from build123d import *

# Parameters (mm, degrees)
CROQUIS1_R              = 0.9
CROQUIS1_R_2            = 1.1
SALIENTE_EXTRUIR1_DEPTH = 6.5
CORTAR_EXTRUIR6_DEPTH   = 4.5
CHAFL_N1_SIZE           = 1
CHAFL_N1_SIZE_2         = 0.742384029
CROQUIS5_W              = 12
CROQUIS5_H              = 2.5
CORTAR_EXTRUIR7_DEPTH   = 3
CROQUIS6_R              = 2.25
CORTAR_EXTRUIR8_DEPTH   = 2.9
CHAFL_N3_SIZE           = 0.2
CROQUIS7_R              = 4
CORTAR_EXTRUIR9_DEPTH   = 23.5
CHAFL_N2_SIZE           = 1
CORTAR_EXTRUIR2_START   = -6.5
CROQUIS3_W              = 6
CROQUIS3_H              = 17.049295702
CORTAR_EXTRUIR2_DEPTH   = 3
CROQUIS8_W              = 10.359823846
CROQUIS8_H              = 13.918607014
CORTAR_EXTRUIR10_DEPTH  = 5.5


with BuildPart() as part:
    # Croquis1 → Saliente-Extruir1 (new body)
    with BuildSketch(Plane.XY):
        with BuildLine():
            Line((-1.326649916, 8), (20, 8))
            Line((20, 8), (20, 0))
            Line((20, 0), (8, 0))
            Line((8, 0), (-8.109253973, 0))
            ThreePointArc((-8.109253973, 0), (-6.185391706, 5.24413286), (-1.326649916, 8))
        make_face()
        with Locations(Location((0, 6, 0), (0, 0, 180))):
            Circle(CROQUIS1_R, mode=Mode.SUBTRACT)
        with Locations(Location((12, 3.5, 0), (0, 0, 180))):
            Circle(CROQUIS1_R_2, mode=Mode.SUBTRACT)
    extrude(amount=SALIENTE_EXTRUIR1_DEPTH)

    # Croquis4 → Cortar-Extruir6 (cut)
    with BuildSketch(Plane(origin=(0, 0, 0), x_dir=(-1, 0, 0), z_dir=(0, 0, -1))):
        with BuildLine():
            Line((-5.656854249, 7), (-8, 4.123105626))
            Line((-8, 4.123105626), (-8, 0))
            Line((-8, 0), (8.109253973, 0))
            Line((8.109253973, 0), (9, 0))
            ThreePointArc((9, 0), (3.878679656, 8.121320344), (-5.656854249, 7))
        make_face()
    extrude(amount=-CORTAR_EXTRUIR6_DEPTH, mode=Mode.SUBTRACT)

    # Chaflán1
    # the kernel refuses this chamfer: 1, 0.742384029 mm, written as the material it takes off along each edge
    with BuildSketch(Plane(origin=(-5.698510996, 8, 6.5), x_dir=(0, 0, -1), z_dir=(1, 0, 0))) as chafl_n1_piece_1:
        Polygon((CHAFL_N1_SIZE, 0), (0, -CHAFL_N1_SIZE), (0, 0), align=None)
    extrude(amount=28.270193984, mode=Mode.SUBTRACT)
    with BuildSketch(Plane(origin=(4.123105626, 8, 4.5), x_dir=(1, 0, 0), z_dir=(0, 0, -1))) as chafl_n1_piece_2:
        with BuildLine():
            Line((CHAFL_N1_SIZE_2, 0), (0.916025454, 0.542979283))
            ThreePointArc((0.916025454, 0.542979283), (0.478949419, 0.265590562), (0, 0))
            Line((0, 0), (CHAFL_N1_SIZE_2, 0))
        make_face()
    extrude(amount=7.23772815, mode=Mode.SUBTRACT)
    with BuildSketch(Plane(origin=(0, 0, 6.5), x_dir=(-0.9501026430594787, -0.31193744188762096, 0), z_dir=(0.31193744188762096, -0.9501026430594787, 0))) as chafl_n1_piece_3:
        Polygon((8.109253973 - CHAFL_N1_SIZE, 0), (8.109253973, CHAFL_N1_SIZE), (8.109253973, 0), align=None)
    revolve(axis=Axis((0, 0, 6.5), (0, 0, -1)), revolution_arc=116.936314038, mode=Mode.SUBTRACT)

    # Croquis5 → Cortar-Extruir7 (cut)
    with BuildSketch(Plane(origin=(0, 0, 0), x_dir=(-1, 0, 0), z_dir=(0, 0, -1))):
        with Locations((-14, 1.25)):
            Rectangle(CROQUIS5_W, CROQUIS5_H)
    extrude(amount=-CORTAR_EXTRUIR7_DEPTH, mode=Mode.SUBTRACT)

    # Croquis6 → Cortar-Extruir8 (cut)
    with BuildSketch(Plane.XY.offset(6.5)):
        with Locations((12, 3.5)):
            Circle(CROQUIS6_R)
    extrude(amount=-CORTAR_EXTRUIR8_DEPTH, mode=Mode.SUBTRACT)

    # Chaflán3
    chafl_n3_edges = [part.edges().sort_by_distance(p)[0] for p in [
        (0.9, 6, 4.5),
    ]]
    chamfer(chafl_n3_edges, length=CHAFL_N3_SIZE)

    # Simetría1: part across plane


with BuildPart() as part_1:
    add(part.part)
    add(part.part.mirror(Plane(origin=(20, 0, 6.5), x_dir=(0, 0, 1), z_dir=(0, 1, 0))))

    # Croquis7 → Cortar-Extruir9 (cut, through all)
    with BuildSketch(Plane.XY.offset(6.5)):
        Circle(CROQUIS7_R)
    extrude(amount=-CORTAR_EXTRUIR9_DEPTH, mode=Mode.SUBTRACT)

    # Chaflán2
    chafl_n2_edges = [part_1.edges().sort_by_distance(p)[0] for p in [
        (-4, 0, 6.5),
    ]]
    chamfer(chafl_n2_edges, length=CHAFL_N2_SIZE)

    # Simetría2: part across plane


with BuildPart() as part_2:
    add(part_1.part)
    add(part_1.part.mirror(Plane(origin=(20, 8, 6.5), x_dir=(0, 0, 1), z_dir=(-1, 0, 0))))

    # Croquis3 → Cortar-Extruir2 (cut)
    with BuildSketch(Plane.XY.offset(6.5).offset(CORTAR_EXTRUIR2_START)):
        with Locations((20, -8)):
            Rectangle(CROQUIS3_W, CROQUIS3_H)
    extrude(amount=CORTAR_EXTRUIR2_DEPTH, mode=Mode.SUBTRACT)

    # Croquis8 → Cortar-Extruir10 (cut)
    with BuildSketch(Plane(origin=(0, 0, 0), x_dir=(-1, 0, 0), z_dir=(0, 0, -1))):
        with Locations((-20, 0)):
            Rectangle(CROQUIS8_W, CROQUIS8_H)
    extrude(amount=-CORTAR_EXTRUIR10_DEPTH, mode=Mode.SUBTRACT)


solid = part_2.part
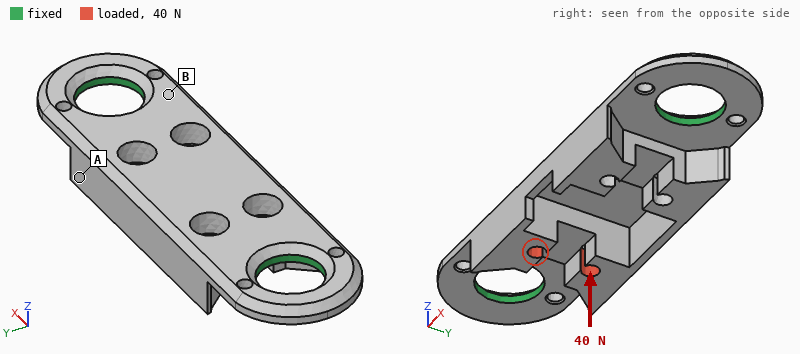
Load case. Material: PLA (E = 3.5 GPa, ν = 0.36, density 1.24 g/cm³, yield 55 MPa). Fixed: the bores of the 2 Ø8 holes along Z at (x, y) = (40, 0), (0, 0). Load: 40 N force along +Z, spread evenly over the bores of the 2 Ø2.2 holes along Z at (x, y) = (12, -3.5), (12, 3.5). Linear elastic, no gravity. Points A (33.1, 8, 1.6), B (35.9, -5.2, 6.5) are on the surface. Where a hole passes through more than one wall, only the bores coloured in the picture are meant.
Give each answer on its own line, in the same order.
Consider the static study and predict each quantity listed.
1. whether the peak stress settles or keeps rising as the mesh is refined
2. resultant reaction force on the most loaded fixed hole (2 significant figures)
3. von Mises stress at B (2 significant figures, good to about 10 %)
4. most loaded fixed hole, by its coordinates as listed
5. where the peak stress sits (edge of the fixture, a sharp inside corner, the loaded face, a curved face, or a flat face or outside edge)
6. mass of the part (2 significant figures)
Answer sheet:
keeps rising
32 N
3.1 MPa
(0, 0)
edge of the fixture
2.4 g
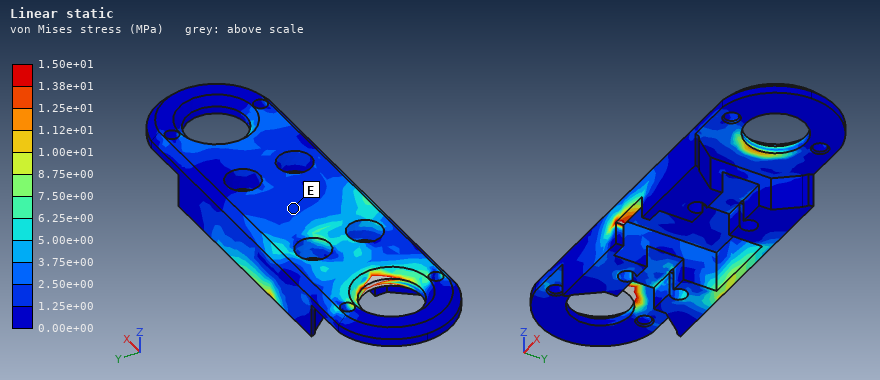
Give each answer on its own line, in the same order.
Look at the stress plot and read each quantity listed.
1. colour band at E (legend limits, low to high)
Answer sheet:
1.25e+00 to 2.50e+00 MPa
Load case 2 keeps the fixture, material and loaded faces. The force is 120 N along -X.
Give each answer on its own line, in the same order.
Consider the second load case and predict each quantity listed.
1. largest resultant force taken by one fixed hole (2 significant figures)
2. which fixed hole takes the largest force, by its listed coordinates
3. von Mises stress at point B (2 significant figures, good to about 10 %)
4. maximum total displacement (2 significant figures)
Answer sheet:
84 N
(0, 0)
3.9 MPa
0.15 mm
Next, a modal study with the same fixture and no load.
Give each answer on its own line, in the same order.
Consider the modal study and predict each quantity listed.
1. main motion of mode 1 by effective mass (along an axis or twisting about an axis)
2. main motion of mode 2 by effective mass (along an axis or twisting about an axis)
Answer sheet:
along Z
along Z
